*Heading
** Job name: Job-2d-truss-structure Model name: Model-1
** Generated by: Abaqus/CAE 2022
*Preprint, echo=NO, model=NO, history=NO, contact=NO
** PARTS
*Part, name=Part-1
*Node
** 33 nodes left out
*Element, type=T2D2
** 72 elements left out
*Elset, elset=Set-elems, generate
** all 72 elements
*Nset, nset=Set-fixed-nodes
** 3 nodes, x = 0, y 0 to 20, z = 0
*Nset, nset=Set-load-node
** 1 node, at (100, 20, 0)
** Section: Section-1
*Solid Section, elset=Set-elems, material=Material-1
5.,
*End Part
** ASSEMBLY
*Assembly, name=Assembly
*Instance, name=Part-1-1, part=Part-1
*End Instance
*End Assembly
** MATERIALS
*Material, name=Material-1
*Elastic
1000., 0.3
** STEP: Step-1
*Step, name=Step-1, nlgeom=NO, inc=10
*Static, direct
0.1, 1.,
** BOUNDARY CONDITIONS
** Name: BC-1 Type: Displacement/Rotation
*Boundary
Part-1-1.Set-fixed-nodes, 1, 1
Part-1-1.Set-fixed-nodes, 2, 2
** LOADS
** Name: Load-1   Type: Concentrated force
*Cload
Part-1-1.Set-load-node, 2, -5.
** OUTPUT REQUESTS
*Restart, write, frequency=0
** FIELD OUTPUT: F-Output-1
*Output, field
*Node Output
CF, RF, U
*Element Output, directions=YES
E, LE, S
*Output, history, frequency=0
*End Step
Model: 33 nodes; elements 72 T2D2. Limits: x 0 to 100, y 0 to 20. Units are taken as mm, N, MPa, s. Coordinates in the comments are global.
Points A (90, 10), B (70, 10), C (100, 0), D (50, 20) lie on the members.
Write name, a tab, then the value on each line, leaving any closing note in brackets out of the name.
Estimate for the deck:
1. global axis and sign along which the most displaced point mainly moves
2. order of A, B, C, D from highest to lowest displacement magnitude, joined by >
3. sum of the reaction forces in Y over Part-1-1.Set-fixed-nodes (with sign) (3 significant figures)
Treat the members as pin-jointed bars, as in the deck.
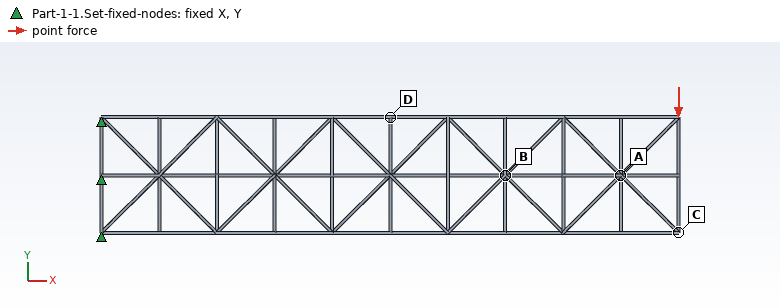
global axis and sign along which the most displaced point mainly moves	-Y
order of A, B, C, D from highest to lowest displacement magnitude, joined by >	C > A > B > D
sum of the reaction forces in Y over Part-1-1.Set-fixed-nodes (with sign)	5.00 N
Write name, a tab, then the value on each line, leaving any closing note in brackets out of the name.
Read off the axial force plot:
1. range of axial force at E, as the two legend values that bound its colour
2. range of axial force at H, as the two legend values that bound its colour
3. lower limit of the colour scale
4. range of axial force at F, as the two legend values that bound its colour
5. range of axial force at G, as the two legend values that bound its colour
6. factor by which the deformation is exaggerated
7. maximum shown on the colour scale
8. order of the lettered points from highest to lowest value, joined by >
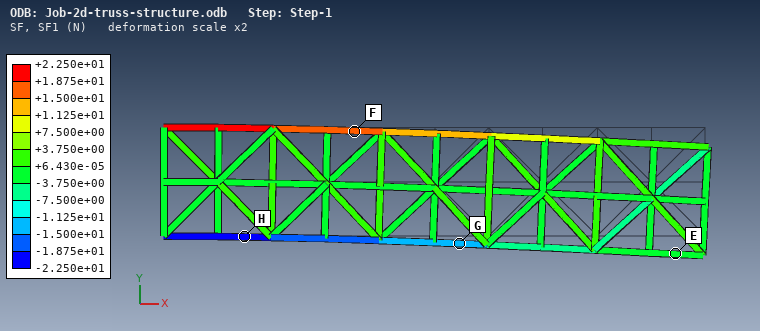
range of axial force at E, as the two legend values that bound its colour	-3.750e+00 to +6.430e-05 N
range of axial force at H, as the two legend values that bound its colour	-2.250e+01 to -1.875e+01 N
lower limit of the colour scale	-2.250e+01 N
range of axial force at F, as the two legend values that bound its colour	+1.500e+01 to +1.875e+01 N
range of axial force at G, as the two legend values that bound its colour	-1.500e+01 to -1.125e+01 N
factor by which the deformation is exaggerated	2
maximum shown on the colour scale	+2.250e+01 N
order of the lettered points from highest to lowest value, joined by >	F > E > G > H
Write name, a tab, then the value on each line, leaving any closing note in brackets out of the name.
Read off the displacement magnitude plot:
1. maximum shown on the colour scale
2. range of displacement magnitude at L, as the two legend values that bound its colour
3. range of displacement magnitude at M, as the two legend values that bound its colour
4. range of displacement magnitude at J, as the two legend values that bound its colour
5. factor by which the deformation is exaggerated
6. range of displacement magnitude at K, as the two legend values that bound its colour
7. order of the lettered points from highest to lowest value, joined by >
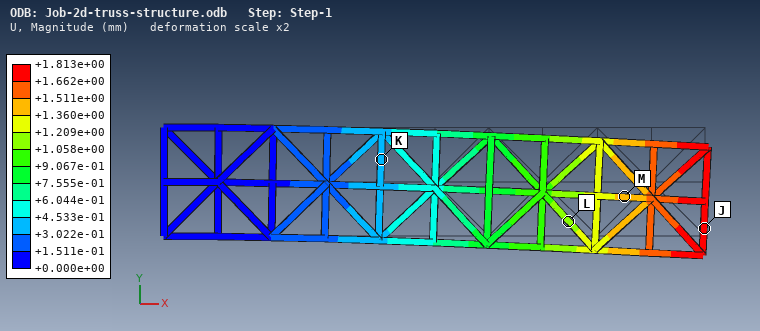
maximum shown on the colour scale	+1.813e+00 mm
range of displacement magnitude at L, as the two legend values that bound its colour	+1.058e+00 to +1.209e+00 mm
range of displacement magnitude at M, as the two legend values that bound its colour	+1.360e+00 to +1.511e+00 mm
range of displacement magnitude at J, as the two legend values that bound its colour	+1.662e+00 to +1.813e+00 mm
factor by which the deformation is exaggerated	2
range of displacement magnitude at K, as the two legend values that bound its colour	+3.022e-01 to +4.533e-01 mm
order of the lettered points from highest to lowest value, joined by >	J > M > L > K
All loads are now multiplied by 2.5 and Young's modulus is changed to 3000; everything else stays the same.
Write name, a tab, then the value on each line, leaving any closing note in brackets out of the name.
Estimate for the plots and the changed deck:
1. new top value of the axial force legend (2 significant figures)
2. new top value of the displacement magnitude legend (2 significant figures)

new top value of the axial force legend	56 N
new top value of the displacement magnitude legend	1.5 mm
